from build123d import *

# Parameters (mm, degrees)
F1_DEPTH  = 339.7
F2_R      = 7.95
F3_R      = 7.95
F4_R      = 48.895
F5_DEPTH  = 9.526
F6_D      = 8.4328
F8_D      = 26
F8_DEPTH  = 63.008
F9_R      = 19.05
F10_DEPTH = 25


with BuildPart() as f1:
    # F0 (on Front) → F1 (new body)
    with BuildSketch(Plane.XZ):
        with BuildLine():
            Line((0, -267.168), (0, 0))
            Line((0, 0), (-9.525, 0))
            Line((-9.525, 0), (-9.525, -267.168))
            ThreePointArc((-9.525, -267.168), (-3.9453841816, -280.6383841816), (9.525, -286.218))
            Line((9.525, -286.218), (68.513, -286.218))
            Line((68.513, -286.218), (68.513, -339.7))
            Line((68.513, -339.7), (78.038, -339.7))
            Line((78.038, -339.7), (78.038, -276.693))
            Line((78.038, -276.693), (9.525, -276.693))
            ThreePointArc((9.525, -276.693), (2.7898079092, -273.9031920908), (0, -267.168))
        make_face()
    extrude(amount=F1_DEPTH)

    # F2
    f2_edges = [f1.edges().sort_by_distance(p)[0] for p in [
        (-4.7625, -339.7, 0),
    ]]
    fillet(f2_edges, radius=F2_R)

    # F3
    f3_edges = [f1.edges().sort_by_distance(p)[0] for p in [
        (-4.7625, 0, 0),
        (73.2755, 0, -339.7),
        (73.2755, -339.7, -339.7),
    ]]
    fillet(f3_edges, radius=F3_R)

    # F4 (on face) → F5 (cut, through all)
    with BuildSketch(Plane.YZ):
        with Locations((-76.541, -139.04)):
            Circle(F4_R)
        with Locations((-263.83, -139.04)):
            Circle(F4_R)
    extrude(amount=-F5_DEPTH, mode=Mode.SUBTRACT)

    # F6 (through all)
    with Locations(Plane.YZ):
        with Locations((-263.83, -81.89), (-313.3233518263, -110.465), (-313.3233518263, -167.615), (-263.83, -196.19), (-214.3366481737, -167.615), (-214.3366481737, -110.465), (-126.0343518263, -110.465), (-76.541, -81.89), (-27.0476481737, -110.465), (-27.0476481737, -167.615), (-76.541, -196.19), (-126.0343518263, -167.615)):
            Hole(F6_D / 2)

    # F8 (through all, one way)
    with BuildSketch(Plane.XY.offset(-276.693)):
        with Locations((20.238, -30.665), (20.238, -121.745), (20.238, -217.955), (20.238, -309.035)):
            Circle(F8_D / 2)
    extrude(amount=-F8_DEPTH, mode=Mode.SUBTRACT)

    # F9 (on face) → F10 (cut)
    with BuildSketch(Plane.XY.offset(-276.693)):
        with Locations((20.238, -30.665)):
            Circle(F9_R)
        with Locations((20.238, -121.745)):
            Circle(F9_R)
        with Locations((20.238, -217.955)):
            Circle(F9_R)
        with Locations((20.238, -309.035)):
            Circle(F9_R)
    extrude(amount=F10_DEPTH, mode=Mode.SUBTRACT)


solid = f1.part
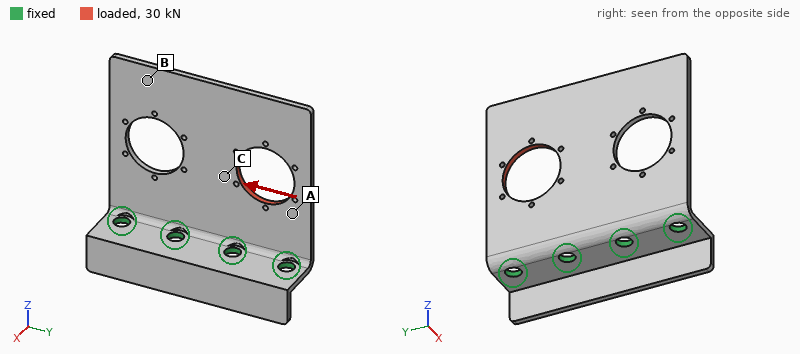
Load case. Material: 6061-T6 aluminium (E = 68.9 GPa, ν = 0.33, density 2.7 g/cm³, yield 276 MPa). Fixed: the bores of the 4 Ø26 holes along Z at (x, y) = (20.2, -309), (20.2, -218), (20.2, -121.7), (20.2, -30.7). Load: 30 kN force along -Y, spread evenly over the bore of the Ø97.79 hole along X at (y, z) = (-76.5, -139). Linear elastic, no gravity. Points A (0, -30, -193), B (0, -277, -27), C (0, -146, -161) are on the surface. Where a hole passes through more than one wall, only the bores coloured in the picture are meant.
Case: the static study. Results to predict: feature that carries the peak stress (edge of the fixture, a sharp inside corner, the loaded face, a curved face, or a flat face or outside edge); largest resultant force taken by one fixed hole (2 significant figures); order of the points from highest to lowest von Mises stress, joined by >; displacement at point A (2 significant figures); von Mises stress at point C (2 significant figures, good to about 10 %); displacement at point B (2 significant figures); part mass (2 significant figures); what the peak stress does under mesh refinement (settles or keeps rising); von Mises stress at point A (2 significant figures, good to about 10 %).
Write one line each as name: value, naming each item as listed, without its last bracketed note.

feature that carries the peak stress: edge of the fixture
largest resultant force taken by one fixed hole: 16 kN
order of the points from highest to lowest von Mises stress, joined by >: C > A > B
displacement at point A: 0.34 mm
von Mises stress at point C: 35 MPa
displacement at point B: 0.48 mm
part mass: 3.1 kg
what the peak stress does under mesh refinement: keeps rising
von Mises stress at point A: 21 MPa
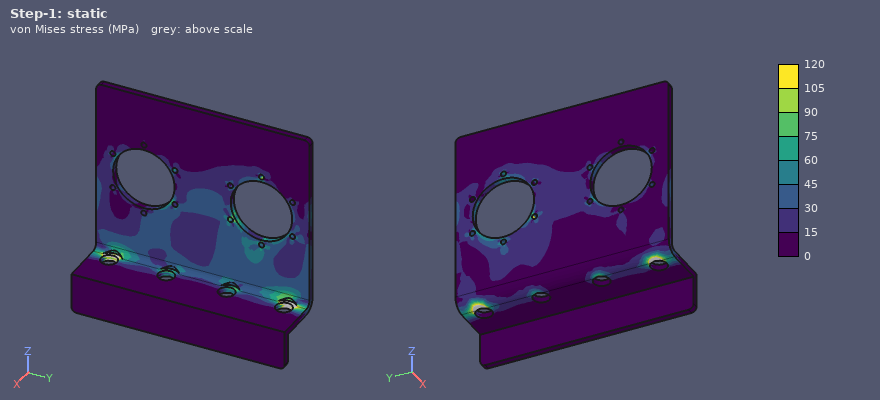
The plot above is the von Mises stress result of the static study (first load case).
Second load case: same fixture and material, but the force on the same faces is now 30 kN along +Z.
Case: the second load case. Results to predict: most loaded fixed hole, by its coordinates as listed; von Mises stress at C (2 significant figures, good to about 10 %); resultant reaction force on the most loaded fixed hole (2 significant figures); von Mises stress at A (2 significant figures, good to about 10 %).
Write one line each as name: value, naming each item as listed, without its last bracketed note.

most loaded fixed hole, by its coordinates as listed: (20.2, -30.7)
von Mises stress at C: 17 MPa
resultant reaction force on the most loaded fixed hole: 16 kN
von Mises stress at A: 28 MPa
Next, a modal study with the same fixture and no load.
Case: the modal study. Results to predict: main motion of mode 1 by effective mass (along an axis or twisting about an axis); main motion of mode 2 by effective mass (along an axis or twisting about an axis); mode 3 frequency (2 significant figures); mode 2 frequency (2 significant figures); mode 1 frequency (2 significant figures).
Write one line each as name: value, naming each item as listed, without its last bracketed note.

main motion of mode 1 by effective mass: along X
main motion of mode 2 by effective mass: twisting about Z
mode 3 frequency: 500 Hz
mode 2 frequency: 190 Hz
mode 1 frequency: 88 Hz
